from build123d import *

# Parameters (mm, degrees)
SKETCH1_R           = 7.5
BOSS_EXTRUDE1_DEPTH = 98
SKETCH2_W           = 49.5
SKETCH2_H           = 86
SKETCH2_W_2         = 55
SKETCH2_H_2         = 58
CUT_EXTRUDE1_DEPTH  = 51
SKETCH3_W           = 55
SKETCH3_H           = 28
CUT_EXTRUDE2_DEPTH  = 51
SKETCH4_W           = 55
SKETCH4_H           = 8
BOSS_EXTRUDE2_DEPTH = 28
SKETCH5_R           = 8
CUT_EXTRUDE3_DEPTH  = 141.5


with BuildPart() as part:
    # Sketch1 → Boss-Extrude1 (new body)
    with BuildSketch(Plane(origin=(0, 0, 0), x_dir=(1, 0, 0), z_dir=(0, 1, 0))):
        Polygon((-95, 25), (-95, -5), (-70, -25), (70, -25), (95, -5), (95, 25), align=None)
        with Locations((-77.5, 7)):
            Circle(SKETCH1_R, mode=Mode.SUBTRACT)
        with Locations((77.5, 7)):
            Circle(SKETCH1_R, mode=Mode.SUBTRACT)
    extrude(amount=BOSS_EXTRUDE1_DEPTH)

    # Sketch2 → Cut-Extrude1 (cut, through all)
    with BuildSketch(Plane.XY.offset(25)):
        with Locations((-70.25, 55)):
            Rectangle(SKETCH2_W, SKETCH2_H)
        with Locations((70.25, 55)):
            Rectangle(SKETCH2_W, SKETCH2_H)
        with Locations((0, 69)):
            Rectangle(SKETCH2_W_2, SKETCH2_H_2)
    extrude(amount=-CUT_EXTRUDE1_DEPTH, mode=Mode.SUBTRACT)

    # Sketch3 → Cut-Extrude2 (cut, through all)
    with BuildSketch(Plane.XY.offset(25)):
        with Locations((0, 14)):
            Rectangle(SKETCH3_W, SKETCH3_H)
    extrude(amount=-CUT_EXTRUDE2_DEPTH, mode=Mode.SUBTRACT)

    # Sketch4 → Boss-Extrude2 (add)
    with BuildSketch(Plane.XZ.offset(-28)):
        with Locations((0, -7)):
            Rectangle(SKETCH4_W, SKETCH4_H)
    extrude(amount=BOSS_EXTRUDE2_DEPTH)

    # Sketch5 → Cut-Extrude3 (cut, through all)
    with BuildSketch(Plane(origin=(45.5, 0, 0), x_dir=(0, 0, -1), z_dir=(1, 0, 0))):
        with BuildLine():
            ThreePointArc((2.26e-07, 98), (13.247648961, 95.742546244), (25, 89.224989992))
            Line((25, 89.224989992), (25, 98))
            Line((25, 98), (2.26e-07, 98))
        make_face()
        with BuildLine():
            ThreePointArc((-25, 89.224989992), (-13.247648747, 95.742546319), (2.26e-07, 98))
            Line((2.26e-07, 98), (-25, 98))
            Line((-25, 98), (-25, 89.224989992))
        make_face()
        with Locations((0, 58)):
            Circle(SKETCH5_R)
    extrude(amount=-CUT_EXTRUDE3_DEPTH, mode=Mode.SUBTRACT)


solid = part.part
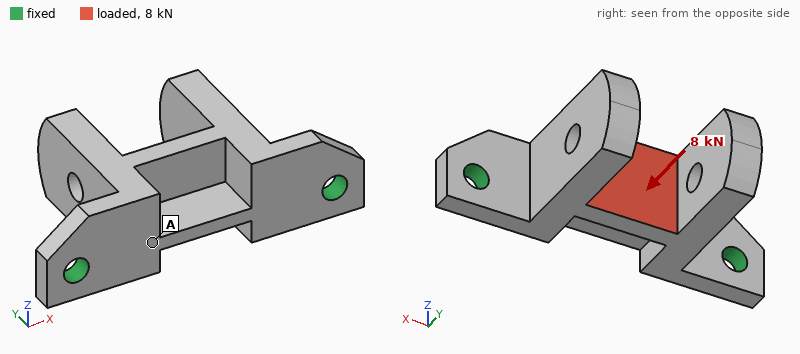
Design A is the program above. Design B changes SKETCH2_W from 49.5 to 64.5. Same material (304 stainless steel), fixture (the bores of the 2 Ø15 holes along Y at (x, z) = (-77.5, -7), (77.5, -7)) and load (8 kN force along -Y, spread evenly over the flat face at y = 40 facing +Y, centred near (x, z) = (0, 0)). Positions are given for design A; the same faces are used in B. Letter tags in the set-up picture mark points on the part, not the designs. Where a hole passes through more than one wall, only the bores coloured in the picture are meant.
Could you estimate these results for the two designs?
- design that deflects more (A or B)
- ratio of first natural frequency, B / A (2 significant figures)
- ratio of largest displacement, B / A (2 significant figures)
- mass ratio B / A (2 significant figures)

B
1.1
1.3
0.77
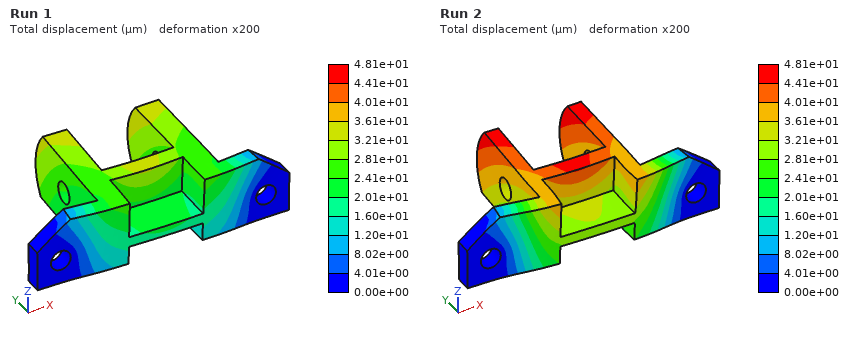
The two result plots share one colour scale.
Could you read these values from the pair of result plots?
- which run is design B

Run 2
